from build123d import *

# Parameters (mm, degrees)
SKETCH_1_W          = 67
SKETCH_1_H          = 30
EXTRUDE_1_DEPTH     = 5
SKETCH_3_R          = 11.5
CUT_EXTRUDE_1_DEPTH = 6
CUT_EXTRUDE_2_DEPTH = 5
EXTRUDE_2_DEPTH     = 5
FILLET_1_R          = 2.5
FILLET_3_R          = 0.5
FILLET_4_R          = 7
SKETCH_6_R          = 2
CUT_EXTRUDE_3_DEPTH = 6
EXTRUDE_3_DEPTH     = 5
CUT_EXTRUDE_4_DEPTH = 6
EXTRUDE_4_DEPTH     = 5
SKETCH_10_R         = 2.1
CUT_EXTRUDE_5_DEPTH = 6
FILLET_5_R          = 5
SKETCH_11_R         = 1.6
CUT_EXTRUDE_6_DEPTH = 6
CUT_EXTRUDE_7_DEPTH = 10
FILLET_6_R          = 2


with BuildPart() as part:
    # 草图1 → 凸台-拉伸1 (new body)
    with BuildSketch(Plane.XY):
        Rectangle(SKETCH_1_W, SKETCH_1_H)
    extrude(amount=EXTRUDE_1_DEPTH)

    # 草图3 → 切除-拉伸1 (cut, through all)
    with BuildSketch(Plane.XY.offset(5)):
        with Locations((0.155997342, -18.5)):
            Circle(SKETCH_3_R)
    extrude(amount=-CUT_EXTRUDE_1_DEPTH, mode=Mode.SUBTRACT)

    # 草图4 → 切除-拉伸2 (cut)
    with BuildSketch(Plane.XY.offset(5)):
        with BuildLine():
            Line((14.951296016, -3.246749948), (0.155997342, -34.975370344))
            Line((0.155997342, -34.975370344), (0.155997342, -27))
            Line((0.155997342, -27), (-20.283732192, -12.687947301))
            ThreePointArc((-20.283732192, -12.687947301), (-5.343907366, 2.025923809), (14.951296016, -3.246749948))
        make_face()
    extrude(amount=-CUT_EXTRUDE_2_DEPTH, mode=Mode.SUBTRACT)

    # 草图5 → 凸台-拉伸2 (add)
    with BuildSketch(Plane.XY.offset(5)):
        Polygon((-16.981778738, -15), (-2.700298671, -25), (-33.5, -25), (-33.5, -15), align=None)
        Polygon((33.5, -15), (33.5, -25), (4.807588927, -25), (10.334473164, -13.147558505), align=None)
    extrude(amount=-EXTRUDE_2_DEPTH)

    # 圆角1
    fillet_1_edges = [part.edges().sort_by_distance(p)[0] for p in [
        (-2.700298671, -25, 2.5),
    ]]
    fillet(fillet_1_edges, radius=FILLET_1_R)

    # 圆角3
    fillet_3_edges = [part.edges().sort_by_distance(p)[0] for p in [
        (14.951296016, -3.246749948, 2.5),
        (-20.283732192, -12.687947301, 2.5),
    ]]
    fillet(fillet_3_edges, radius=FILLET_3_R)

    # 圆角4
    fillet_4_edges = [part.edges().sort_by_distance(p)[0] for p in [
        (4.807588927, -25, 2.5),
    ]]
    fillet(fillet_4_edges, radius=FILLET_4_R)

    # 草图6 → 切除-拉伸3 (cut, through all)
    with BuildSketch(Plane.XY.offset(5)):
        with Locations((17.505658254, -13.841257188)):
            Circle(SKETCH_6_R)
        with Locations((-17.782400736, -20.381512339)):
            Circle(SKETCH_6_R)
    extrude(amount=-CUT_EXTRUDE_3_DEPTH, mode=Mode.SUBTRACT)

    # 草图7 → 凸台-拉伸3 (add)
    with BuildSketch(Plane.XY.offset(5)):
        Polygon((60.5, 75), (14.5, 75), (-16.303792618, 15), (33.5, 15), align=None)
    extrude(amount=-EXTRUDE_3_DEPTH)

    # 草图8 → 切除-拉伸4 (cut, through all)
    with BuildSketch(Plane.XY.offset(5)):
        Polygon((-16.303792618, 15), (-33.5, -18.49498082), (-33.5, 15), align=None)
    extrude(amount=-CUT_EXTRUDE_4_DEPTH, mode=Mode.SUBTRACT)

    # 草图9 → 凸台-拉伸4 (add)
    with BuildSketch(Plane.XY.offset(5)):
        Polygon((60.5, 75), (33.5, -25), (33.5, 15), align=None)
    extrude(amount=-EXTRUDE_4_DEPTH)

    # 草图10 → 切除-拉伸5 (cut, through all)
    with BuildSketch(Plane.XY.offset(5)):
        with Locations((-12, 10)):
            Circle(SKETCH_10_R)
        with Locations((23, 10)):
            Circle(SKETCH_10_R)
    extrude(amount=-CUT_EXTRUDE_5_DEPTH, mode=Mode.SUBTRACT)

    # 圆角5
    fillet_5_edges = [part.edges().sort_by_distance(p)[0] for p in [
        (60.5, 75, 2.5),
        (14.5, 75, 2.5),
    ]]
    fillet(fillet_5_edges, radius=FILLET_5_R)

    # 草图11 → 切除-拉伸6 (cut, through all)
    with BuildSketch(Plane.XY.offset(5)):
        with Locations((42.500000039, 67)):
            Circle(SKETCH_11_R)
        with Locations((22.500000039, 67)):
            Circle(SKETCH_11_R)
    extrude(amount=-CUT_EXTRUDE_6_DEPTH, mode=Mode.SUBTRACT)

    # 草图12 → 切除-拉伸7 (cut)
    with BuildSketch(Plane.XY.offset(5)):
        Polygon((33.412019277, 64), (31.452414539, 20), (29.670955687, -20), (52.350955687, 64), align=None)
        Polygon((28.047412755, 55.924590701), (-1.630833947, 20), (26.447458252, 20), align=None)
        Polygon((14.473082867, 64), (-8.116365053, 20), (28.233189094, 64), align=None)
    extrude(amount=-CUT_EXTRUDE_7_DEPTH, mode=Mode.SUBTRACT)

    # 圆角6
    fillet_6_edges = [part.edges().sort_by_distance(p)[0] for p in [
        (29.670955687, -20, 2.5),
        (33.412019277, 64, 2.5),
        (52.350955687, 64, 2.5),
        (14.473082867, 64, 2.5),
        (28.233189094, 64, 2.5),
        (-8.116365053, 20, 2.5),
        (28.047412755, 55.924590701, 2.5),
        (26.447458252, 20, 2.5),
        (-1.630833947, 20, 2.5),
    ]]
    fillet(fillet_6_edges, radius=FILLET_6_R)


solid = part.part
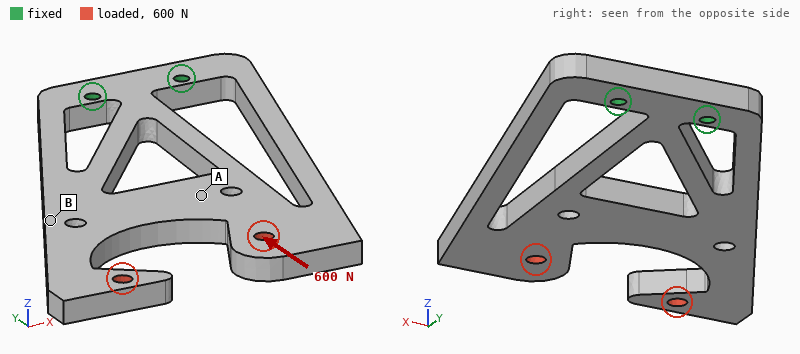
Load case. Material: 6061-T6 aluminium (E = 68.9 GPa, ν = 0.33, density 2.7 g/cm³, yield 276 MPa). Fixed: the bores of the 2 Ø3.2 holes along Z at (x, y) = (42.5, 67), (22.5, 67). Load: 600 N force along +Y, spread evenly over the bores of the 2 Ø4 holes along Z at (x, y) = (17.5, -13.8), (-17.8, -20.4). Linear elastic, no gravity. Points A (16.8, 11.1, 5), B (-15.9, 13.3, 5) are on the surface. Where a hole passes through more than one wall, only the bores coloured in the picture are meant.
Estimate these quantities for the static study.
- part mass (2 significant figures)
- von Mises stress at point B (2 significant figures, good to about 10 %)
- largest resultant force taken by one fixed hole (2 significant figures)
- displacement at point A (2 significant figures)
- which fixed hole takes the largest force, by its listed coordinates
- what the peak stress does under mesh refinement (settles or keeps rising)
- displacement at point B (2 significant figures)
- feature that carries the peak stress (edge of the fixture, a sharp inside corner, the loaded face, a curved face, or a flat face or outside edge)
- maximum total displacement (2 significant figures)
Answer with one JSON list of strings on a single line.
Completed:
["47 g", "11 MPa", "1.1 kN", "0.10 mm", "(22.5, 67)", "keeps rising", "0.12 mm", "edge of the fixture", "0.18 mm"]
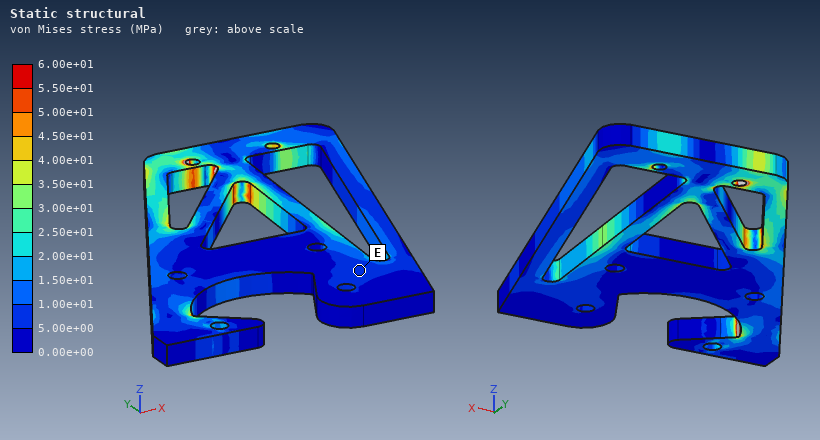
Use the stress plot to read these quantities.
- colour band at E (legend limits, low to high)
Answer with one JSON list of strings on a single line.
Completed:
["5.00e+00 to 1.00e+01 MPa"]
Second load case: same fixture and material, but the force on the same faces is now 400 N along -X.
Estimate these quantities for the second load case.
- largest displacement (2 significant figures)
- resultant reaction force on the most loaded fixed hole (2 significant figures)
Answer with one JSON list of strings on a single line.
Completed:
["0.45 mm", "1.4 kN"]
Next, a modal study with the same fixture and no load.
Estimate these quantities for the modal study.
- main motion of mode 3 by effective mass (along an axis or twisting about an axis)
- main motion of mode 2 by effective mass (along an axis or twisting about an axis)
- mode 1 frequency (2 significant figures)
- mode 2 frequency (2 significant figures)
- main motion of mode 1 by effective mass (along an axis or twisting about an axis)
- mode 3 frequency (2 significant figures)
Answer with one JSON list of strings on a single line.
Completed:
["along X", "twisting about Y", "280 Hz", "760 Hz", "along Z", "1200 Hz"]
